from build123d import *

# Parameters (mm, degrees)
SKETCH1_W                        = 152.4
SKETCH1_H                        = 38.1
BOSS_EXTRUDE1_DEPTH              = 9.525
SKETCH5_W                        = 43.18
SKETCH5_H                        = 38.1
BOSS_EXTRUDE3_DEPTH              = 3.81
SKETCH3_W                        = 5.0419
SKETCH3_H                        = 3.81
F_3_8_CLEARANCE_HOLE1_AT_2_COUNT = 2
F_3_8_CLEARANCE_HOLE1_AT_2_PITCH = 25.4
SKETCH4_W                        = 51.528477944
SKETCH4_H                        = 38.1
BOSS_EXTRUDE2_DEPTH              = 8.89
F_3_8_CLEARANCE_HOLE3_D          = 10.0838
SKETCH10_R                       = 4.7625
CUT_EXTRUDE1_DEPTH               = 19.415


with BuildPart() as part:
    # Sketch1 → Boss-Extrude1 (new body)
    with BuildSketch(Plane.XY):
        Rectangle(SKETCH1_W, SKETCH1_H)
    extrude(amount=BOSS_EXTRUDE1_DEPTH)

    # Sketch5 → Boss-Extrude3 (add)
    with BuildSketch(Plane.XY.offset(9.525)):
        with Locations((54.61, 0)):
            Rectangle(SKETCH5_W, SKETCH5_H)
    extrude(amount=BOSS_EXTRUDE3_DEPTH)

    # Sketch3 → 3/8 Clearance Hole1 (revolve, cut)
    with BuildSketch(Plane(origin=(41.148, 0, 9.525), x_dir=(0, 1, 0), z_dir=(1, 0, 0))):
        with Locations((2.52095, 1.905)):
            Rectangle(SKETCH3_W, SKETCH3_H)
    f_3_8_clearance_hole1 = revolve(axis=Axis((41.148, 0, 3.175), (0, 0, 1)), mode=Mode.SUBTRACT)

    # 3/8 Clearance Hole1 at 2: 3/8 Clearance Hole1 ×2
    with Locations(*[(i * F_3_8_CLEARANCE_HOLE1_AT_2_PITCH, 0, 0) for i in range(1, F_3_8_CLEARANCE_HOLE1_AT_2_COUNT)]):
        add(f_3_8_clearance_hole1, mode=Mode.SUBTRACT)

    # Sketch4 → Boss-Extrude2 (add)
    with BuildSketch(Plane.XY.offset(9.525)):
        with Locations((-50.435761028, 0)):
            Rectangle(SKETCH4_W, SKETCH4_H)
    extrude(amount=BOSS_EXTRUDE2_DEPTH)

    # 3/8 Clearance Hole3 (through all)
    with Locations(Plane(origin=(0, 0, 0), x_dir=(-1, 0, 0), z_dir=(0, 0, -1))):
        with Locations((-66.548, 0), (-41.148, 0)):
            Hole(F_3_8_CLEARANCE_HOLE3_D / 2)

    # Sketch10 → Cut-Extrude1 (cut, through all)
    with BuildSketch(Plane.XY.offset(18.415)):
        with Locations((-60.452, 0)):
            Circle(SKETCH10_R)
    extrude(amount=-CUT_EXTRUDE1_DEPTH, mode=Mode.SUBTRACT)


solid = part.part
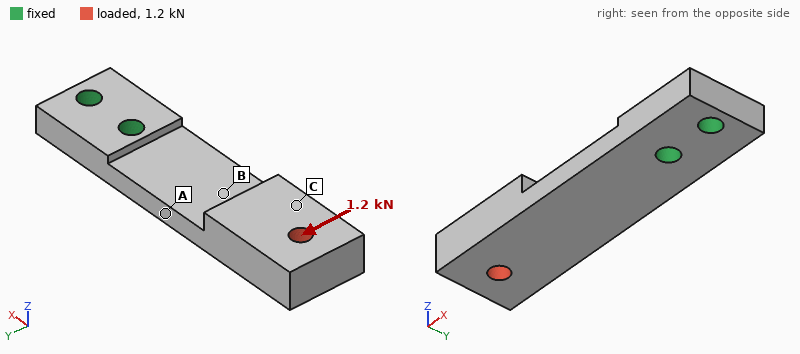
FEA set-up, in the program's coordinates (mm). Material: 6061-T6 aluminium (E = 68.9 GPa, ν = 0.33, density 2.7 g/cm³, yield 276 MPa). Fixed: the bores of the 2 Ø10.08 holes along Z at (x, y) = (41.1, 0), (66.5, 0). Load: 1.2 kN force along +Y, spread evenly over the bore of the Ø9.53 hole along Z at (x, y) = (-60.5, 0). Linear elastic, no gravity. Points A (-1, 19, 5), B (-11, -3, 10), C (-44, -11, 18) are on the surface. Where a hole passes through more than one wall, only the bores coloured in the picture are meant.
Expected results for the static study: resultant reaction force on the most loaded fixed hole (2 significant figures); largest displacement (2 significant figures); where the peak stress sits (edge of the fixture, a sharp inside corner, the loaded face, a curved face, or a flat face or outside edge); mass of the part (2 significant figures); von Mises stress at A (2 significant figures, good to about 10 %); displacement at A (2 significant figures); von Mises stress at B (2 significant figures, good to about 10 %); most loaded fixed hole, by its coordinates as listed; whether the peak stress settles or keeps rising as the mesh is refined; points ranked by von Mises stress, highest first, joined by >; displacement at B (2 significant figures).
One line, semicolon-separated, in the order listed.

3.8 kN; 0.25 mm; edge of the fixture; 200 g; 32 MPa; 0.065 mm; 16 MPa; (41.1, 0); keeps rising; A > B > C; 0.077 mm
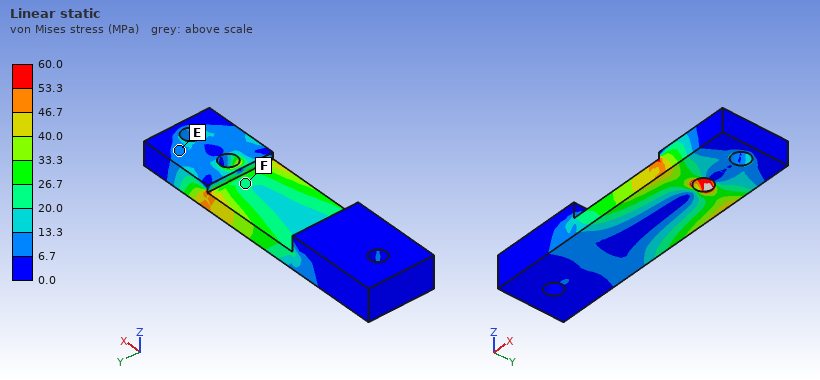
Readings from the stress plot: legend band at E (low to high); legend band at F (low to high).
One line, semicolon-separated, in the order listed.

6.7 to 13.3 MPa; 20.0 to 26.7 MPa
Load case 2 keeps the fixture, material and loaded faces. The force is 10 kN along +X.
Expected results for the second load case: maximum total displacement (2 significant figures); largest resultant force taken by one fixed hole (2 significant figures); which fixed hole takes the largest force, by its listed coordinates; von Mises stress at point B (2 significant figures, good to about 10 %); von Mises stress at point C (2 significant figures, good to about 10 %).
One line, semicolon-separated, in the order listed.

1.2 mm; 8.2 kN; (41.1, 0); 100 MPa; 15 MPa
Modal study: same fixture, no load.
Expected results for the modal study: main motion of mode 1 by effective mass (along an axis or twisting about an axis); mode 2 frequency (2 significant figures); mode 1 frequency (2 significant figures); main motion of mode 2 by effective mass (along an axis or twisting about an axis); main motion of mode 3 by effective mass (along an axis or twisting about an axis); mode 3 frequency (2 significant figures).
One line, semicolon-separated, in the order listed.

along Z; 1400 Hz; 460 Hz; along Y; twisting about X; 2600 Hz
